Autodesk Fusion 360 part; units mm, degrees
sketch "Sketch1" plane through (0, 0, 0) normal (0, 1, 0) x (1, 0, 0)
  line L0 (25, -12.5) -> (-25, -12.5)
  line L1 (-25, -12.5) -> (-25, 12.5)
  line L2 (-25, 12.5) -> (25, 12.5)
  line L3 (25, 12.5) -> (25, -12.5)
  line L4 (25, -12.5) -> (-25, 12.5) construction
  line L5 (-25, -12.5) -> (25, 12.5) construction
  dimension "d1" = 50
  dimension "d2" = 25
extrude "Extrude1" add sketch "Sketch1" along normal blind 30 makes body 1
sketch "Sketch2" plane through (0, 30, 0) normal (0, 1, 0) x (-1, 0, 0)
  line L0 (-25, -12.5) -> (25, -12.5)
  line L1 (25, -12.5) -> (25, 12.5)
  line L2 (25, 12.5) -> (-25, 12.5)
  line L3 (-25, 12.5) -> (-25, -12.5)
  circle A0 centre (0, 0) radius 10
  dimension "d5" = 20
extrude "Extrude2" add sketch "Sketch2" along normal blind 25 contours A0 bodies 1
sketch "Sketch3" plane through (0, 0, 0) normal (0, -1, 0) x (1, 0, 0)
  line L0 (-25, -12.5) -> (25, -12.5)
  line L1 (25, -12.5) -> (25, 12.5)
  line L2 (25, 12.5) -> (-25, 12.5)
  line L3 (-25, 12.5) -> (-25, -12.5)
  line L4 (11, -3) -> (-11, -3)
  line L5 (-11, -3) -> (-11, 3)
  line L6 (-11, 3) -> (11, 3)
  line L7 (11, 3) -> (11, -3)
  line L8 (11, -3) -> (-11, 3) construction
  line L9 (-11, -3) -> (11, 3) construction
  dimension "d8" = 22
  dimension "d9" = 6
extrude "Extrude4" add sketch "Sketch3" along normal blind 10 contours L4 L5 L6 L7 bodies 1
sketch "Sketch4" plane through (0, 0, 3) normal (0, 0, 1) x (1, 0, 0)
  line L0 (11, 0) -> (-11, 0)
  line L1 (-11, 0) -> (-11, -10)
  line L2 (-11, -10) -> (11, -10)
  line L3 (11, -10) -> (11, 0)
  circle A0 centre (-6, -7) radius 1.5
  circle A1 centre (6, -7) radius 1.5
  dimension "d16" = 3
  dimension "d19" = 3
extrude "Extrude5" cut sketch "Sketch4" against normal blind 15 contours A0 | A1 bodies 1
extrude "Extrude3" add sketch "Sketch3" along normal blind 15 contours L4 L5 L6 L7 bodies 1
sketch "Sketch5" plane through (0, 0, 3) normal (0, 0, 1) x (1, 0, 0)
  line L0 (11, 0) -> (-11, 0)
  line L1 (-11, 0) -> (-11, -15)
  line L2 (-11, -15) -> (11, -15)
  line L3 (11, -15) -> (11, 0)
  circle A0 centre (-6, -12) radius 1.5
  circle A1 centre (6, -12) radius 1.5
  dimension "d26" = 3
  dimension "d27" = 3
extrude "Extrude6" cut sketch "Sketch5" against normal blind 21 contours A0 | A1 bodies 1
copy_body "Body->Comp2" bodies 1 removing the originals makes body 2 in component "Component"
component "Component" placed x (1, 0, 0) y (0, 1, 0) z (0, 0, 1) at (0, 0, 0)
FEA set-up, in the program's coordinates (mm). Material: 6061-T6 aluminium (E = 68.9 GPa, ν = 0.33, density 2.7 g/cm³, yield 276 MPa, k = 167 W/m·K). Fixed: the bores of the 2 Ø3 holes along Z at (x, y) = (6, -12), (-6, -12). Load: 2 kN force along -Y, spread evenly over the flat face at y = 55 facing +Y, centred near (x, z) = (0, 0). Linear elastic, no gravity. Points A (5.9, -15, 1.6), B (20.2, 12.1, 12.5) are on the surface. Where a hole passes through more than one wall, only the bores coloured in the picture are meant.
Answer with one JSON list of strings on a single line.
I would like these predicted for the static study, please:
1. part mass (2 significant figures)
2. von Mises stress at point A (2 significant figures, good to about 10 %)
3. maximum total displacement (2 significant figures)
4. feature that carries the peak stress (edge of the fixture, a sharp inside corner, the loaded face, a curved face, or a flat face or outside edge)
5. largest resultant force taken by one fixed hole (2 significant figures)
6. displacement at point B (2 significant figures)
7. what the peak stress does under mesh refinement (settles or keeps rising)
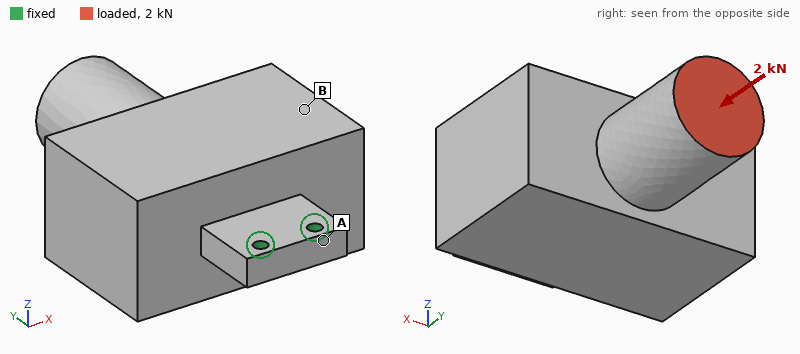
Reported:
["130 g", "12 MPa", "7.3 µm", "edge of the fixture", "1.0 kN", "4.1 µm", "keeps rising"]
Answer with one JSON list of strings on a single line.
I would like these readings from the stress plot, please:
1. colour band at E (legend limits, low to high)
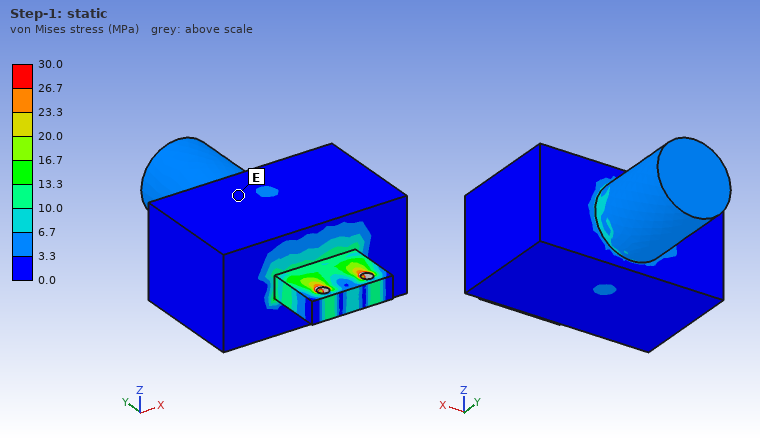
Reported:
["0.0 to 3.3 MPa"]
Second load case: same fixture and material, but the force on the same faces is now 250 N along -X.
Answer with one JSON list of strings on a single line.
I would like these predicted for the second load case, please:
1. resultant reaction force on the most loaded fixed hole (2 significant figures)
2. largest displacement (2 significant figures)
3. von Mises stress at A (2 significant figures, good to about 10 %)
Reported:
["1.2 kN", "51 µm", "16 MPa"]
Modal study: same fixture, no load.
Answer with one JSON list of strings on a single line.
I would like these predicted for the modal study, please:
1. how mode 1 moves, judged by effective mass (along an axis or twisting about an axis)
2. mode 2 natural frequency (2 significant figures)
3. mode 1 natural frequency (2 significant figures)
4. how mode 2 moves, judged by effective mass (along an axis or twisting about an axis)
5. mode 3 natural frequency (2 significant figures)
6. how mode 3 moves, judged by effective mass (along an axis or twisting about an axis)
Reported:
["along Z", "2000 Hz", "690 Hz", "along X", "2200 Hz", "twisting about Y"]
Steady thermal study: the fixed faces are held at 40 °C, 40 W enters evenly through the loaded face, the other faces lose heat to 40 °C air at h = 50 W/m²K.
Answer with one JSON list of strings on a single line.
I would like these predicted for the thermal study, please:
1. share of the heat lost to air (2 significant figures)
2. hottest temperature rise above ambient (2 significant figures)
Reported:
["26 %", "45 K"]
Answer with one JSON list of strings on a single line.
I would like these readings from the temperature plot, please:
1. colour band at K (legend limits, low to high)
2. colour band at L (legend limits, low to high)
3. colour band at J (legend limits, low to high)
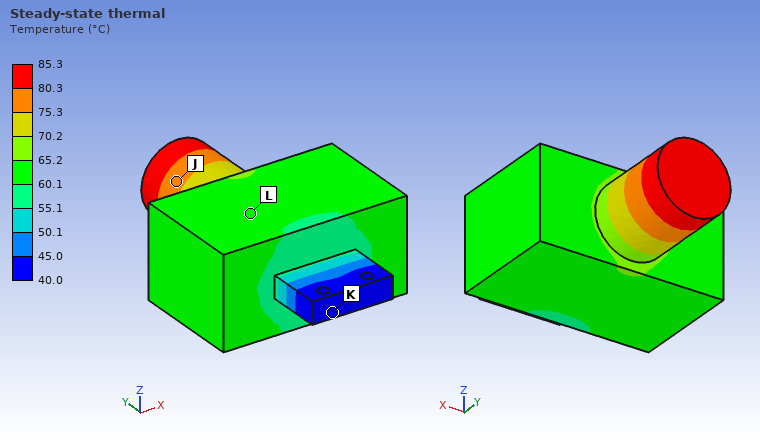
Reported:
["40.0 to 45.0 °C", "60.1 to 65.2 °C", "75.3 to 80.3 °C"]
